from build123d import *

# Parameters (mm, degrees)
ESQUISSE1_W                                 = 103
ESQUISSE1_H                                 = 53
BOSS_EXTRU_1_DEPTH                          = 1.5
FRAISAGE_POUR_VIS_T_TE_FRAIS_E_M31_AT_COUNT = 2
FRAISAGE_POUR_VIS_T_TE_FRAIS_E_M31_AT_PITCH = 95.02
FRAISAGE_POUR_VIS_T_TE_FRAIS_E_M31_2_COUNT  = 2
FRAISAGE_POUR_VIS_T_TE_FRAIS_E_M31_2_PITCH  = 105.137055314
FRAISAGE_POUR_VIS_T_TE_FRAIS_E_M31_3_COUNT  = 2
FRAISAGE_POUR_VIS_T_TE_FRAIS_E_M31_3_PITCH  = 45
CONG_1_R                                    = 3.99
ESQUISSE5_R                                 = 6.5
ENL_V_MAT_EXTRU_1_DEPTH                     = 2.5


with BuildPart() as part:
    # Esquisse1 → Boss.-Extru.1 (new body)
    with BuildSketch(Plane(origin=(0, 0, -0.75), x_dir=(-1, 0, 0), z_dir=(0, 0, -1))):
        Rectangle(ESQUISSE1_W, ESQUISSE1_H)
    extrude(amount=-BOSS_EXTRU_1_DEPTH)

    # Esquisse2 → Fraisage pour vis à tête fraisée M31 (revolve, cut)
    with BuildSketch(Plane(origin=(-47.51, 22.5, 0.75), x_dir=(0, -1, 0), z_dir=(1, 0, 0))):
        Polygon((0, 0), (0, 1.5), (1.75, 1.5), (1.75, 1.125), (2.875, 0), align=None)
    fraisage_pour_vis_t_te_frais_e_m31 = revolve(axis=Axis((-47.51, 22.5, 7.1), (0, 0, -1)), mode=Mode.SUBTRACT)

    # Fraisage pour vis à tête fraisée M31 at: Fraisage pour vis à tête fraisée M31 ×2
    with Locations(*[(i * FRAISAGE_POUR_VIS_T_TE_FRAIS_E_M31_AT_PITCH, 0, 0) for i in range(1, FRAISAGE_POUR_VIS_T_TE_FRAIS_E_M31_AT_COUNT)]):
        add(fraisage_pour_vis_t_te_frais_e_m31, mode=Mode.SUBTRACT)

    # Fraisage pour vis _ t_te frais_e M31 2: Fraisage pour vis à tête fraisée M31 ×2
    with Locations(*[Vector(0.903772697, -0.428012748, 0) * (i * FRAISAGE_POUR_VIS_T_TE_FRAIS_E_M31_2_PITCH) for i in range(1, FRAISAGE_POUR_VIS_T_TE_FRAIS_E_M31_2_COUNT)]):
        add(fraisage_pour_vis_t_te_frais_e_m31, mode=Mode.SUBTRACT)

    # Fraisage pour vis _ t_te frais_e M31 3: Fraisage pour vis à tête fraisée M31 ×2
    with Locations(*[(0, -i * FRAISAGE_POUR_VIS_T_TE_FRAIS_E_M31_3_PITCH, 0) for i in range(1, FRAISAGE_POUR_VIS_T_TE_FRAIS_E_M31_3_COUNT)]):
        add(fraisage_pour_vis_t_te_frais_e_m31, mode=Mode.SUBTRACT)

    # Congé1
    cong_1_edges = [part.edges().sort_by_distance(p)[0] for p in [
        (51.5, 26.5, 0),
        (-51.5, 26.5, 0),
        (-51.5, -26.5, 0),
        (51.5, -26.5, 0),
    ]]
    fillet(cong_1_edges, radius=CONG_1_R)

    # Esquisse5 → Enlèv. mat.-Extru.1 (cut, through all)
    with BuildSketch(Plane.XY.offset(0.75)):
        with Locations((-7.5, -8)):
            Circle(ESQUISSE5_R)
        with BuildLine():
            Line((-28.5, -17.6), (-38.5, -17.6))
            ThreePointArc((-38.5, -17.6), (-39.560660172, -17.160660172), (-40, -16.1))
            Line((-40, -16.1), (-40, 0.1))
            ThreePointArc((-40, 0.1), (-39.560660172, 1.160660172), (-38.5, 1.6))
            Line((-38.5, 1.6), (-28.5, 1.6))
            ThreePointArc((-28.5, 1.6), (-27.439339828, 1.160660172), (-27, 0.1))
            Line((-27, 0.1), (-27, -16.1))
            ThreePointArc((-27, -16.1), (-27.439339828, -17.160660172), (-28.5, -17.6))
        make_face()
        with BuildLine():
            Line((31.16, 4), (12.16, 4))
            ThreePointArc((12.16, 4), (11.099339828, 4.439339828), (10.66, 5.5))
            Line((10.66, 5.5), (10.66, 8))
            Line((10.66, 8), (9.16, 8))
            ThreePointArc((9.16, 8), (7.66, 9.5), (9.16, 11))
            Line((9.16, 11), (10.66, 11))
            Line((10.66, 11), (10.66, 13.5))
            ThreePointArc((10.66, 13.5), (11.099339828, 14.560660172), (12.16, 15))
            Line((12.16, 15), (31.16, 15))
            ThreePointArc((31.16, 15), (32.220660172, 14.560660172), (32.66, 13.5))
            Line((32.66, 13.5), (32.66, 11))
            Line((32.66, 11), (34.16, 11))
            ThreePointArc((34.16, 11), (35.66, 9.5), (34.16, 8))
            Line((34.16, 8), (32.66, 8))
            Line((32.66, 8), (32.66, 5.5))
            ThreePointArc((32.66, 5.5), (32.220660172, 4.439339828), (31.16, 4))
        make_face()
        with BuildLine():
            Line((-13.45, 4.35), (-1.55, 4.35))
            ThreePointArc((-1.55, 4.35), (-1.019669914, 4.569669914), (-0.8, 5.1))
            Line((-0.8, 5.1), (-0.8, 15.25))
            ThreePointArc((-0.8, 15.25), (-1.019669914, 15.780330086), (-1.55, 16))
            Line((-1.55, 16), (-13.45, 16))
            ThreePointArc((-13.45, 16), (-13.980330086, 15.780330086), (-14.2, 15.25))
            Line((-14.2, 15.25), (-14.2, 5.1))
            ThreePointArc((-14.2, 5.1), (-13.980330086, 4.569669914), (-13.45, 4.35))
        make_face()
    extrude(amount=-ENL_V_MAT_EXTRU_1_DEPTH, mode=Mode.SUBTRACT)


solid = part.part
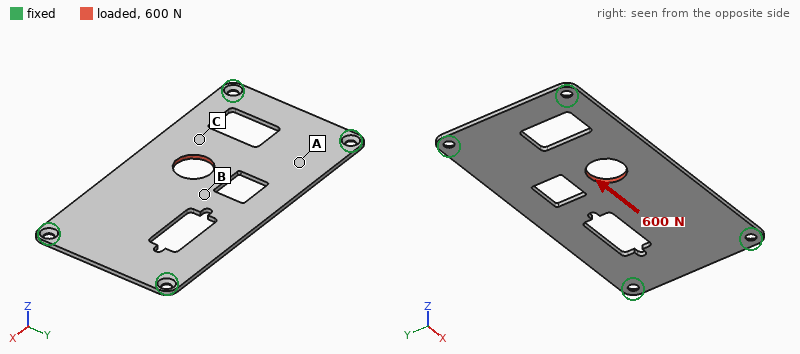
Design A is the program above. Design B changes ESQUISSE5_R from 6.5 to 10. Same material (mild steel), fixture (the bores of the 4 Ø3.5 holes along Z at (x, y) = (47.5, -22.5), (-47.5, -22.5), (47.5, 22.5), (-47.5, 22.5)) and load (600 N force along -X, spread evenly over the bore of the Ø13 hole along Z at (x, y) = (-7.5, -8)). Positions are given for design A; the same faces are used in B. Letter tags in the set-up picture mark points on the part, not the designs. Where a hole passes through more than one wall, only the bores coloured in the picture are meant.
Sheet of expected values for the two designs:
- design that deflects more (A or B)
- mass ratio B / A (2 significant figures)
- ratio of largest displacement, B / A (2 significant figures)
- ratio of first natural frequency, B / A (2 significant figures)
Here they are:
B
0.96
1.1
1.0
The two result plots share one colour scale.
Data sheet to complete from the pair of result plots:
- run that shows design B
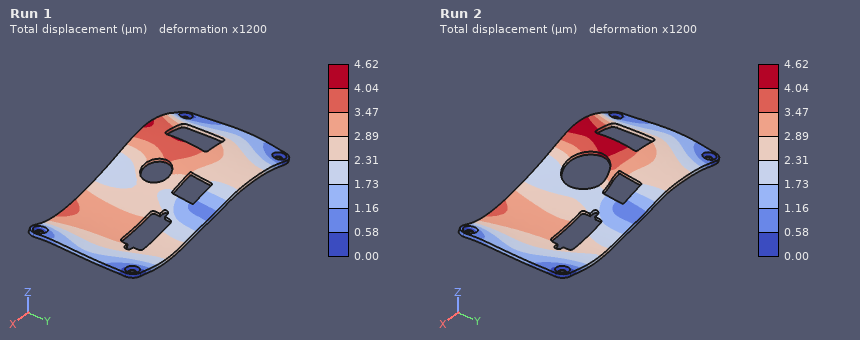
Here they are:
Run 2
